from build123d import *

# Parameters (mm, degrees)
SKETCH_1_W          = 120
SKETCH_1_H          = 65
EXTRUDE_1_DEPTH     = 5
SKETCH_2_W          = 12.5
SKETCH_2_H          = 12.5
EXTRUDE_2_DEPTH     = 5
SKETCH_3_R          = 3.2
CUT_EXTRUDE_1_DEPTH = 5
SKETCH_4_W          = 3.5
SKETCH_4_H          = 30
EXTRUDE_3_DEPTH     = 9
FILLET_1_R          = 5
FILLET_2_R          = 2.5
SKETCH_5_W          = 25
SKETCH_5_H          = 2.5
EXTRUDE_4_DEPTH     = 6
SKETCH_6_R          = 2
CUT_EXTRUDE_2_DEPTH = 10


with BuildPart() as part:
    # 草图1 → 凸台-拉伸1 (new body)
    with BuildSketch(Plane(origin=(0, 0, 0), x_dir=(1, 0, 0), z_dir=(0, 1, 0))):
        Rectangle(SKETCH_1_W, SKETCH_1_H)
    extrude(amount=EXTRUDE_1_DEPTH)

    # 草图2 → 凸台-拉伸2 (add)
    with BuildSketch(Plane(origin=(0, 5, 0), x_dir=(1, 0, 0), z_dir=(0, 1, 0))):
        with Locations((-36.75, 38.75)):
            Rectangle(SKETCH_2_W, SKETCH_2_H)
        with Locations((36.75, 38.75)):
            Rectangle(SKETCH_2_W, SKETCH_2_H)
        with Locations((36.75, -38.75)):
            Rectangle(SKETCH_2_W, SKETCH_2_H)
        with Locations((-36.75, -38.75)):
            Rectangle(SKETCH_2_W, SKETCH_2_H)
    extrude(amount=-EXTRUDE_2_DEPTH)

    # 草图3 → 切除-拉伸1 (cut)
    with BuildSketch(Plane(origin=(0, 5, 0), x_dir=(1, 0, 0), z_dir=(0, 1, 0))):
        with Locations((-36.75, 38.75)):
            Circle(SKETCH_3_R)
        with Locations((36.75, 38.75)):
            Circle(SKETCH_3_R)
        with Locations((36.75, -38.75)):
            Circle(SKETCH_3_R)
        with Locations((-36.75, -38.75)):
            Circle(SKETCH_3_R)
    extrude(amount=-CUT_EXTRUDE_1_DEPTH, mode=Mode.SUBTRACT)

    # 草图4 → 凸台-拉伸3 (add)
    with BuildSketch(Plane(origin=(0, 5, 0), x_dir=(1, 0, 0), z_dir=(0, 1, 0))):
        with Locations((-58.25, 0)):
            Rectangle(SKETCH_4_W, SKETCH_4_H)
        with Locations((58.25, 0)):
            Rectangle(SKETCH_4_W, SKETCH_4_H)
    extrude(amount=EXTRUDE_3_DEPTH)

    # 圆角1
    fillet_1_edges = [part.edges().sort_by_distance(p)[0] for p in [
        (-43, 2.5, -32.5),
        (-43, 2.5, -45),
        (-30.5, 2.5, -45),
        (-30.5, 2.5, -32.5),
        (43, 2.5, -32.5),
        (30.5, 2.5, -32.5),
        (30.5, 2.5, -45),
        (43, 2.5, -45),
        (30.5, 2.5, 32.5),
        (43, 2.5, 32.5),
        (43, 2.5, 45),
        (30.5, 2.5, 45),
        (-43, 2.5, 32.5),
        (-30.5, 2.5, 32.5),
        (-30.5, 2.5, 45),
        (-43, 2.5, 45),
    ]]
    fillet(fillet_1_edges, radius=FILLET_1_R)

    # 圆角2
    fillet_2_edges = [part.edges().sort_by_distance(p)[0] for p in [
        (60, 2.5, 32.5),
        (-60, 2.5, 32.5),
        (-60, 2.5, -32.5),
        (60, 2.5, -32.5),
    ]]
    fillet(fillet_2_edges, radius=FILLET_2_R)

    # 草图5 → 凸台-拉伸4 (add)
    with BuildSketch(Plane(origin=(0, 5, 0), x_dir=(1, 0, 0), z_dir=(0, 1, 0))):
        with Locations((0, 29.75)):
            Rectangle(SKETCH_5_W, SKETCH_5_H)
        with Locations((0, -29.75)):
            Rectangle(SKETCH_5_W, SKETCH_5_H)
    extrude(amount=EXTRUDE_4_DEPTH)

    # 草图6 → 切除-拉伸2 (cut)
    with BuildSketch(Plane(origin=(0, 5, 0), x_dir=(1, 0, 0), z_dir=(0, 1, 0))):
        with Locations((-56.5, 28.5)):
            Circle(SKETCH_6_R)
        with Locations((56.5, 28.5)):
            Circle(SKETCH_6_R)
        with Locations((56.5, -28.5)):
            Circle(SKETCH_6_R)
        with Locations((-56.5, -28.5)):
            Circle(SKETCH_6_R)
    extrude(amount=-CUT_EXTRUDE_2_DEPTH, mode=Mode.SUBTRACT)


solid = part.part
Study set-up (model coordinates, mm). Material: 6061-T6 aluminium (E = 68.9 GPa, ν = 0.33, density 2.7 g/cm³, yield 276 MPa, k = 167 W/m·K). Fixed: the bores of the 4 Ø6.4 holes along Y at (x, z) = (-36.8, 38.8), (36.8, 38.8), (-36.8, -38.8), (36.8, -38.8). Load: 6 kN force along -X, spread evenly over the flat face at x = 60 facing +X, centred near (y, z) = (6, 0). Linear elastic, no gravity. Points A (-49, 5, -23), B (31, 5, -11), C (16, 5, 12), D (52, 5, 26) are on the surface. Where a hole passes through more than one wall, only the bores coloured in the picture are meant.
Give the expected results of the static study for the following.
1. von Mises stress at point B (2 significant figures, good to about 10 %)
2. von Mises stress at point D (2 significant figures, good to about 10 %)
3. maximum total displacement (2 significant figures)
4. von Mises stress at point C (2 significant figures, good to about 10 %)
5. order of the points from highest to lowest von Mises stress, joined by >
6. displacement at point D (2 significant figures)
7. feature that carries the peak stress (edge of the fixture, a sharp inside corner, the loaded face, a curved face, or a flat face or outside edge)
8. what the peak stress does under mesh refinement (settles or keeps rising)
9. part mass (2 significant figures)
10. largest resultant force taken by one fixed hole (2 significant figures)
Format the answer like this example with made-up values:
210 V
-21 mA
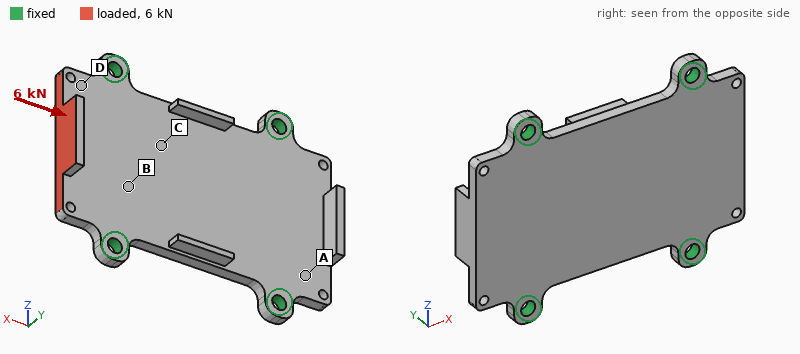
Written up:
53 MPa
77 MPa
0.33 mm
30 MPa
D > B > C > A
0.088 mm
edge of the fixture
keeps rising
120 g
1.9 kN
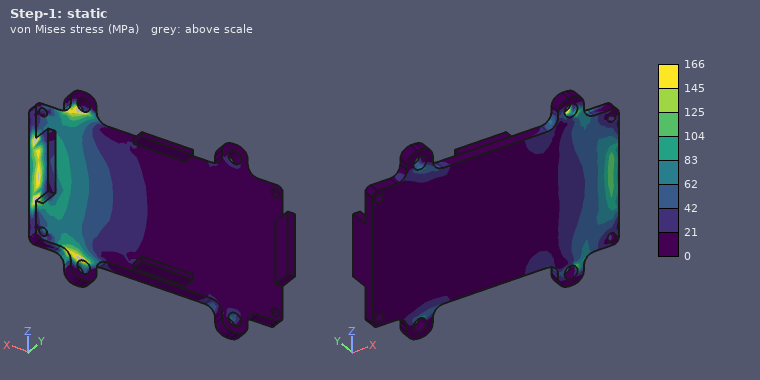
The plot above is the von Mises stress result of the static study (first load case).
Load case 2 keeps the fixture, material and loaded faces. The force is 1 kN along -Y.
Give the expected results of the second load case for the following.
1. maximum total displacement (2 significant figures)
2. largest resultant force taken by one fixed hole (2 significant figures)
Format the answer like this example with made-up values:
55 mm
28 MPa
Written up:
0.29 mm
580 N
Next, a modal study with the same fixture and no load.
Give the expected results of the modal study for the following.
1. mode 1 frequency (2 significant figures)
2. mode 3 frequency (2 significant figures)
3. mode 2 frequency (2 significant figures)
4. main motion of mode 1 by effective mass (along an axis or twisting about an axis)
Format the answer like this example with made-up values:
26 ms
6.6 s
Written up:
3000 Hz
3200 Hz
3200 Hz
along Y
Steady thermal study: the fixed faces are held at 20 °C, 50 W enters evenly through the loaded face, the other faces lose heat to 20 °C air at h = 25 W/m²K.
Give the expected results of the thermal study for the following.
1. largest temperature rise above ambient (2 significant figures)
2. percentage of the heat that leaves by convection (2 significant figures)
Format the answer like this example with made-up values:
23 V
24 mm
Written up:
47 K
10 %
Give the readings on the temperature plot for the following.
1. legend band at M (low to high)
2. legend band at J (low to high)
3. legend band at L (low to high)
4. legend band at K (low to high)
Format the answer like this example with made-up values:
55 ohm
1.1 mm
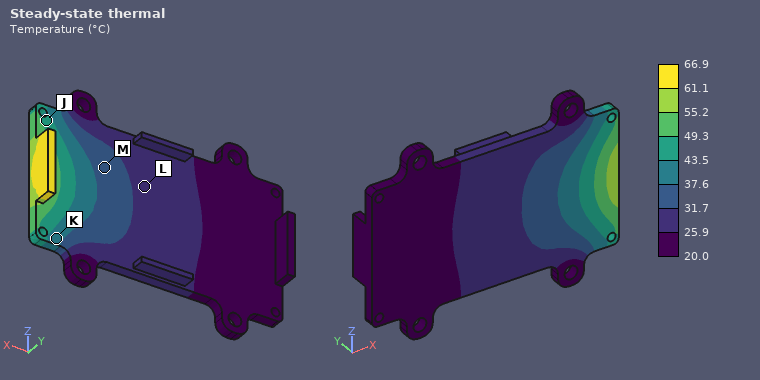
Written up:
31.7 to 37.6 °C
43.5 to 49.3 °C
25.9 to 31.7 °C
37.6 to 43.5 °C
